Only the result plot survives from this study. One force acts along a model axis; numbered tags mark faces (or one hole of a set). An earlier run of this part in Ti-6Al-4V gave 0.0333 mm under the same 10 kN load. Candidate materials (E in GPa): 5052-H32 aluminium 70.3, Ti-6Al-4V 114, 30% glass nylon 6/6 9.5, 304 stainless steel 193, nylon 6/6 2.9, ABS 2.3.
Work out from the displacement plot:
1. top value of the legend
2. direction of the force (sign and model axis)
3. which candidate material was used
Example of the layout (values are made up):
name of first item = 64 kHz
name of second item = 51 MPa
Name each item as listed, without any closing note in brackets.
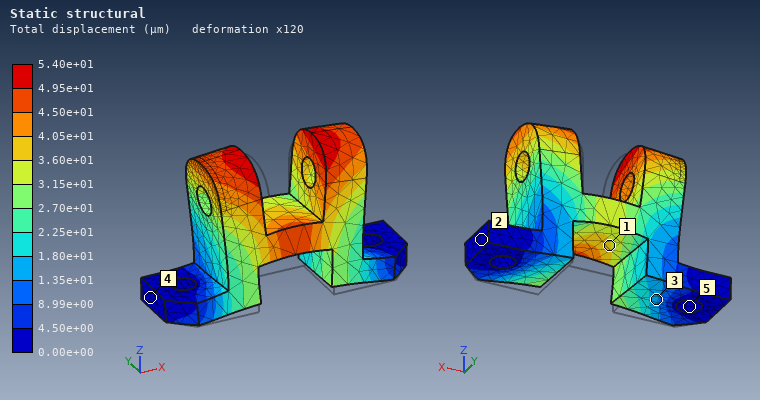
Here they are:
top value of the legend = 5.40e+01 µm
direction of the force = +Z
which candidate material was used = 5052-H32 aluminium
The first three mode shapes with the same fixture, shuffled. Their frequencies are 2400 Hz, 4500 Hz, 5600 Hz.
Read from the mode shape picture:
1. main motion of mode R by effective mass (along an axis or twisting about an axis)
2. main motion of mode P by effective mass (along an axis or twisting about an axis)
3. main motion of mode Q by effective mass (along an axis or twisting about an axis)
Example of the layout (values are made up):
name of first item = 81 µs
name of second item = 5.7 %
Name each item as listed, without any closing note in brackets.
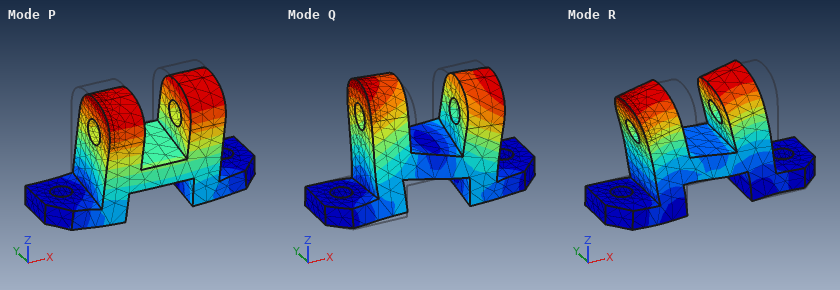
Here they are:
main motion of mode R by effective mass = along X
main motion of mode P by effective mass = along Y
main motion of mode Q by effective mass = twisting about Z
